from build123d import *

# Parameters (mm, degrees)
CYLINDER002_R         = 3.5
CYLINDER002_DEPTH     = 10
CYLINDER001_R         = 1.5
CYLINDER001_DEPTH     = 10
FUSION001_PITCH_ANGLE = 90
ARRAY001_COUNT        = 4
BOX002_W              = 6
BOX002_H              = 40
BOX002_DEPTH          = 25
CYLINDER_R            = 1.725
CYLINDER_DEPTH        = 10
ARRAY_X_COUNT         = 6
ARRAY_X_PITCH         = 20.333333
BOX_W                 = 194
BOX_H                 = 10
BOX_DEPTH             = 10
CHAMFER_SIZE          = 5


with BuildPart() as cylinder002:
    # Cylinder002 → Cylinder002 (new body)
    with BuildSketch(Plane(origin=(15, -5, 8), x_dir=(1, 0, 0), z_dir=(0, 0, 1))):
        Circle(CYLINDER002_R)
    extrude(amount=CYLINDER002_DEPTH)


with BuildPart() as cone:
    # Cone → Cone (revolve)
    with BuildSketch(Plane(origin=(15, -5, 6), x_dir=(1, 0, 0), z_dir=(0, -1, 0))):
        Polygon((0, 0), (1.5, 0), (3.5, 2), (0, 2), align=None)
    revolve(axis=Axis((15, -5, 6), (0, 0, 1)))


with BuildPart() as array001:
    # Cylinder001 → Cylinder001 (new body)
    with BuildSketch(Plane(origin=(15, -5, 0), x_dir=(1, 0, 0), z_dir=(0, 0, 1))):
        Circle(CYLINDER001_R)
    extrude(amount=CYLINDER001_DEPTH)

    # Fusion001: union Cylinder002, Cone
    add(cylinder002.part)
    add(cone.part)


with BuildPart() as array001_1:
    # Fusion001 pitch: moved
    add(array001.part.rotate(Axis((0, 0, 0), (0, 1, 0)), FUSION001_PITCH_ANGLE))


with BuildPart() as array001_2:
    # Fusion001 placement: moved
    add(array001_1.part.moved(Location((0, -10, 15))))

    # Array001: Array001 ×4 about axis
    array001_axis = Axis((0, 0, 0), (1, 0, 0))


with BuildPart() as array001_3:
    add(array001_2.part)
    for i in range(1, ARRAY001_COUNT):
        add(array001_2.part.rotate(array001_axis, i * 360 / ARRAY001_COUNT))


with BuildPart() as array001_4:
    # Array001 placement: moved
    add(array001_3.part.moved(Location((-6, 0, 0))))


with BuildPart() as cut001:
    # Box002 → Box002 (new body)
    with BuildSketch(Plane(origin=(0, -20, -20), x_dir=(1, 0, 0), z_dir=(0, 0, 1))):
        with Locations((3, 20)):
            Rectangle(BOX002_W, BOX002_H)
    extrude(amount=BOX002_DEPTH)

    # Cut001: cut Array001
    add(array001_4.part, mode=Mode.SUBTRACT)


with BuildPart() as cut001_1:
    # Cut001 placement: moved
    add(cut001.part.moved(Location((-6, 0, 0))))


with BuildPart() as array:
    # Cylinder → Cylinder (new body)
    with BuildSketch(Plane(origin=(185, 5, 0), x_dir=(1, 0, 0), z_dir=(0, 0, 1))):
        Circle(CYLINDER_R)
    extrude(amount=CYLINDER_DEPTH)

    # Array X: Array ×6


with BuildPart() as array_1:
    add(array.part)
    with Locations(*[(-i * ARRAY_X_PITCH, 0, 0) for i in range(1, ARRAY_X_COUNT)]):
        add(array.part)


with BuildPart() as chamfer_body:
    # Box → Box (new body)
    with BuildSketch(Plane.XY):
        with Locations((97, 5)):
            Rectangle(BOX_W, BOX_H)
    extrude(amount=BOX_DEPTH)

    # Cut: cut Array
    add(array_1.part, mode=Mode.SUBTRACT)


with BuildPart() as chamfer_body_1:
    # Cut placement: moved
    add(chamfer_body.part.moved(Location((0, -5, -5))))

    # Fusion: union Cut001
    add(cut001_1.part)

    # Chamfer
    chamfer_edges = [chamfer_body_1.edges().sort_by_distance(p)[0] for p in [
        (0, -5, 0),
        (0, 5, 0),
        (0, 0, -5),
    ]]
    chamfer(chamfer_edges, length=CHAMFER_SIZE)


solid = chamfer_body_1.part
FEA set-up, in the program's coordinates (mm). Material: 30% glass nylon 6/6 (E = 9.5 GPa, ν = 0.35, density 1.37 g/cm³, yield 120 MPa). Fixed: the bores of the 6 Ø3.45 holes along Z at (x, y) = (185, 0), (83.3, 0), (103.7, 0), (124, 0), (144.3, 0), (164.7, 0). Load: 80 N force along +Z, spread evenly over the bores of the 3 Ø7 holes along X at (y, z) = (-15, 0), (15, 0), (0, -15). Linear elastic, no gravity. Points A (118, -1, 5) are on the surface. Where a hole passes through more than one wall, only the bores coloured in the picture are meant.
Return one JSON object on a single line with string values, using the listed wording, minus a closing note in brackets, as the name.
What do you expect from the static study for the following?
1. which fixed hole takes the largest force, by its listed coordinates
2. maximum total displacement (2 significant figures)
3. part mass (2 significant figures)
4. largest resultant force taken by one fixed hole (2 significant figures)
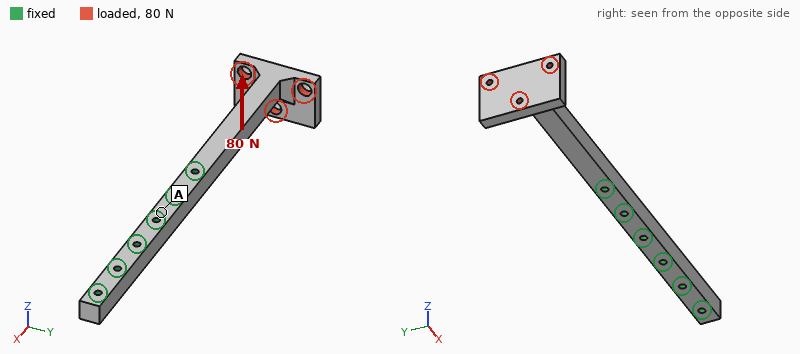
{"which fixed hole takes the largest force, by its listed coordinates": "(83.3, 0)", "maximum total displacement": "2.4 mm", "part mass": "34 g", "largest resultant force taken by one fixed hole": "120 N"}
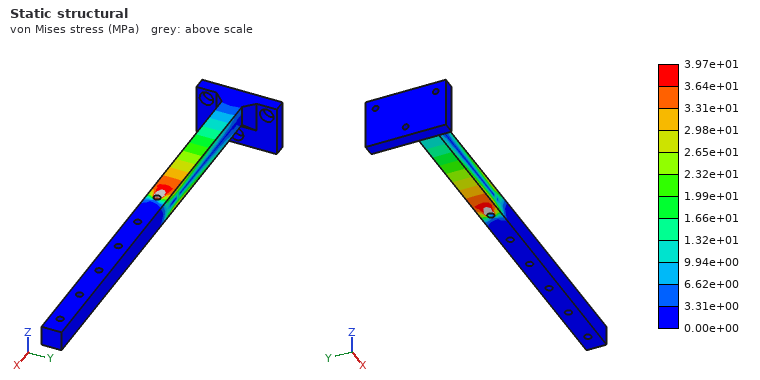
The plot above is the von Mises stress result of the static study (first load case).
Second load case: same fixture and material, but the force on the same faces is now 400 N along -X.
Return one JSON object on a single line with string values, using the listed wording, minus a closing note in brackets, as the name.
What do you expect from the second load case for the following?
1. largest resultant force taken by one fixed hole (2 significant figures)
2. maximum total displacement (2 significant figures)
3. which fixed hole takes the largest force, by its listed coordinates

{"largest resultant force taken by one fixed hole": "380 N", "maximum total displacement": "1.1 mm", "which fixed hole takes the largest force, by its listed coordinates": "(83.3, 0)"}
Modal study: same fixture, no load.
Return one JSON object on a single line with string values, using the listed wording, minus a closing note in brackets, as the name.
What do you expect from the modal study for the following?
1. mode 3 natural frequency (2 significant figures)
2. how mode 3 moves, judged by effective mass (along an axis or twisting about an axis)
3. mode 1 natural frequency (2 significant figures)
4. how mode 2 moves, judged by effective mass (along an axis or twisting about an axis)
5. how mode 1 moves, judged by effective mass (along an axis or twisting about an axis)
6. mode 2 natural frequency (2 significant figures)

{"mode 3 natural frequency": "1000 Hz", "how mode 3 moves, judged by effective mass": "twisting about X", "mode 1 natural frequency": "280 Hz", "how mode 2 moves, judged by effective mass": "along Z", "how mode 1 moves, judged by effective mass": "along Y", "mode 2 natural frequency": "300 Hz"}
